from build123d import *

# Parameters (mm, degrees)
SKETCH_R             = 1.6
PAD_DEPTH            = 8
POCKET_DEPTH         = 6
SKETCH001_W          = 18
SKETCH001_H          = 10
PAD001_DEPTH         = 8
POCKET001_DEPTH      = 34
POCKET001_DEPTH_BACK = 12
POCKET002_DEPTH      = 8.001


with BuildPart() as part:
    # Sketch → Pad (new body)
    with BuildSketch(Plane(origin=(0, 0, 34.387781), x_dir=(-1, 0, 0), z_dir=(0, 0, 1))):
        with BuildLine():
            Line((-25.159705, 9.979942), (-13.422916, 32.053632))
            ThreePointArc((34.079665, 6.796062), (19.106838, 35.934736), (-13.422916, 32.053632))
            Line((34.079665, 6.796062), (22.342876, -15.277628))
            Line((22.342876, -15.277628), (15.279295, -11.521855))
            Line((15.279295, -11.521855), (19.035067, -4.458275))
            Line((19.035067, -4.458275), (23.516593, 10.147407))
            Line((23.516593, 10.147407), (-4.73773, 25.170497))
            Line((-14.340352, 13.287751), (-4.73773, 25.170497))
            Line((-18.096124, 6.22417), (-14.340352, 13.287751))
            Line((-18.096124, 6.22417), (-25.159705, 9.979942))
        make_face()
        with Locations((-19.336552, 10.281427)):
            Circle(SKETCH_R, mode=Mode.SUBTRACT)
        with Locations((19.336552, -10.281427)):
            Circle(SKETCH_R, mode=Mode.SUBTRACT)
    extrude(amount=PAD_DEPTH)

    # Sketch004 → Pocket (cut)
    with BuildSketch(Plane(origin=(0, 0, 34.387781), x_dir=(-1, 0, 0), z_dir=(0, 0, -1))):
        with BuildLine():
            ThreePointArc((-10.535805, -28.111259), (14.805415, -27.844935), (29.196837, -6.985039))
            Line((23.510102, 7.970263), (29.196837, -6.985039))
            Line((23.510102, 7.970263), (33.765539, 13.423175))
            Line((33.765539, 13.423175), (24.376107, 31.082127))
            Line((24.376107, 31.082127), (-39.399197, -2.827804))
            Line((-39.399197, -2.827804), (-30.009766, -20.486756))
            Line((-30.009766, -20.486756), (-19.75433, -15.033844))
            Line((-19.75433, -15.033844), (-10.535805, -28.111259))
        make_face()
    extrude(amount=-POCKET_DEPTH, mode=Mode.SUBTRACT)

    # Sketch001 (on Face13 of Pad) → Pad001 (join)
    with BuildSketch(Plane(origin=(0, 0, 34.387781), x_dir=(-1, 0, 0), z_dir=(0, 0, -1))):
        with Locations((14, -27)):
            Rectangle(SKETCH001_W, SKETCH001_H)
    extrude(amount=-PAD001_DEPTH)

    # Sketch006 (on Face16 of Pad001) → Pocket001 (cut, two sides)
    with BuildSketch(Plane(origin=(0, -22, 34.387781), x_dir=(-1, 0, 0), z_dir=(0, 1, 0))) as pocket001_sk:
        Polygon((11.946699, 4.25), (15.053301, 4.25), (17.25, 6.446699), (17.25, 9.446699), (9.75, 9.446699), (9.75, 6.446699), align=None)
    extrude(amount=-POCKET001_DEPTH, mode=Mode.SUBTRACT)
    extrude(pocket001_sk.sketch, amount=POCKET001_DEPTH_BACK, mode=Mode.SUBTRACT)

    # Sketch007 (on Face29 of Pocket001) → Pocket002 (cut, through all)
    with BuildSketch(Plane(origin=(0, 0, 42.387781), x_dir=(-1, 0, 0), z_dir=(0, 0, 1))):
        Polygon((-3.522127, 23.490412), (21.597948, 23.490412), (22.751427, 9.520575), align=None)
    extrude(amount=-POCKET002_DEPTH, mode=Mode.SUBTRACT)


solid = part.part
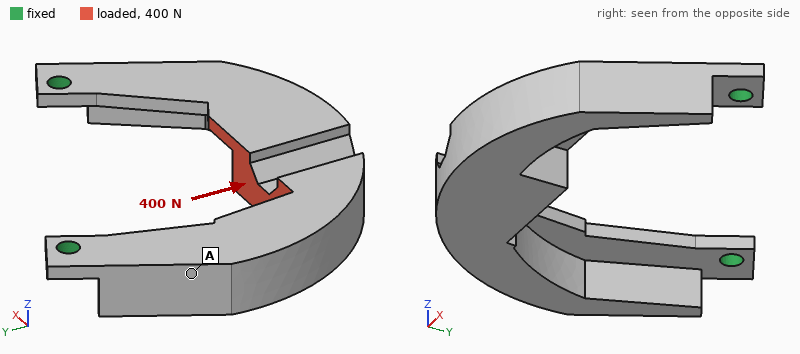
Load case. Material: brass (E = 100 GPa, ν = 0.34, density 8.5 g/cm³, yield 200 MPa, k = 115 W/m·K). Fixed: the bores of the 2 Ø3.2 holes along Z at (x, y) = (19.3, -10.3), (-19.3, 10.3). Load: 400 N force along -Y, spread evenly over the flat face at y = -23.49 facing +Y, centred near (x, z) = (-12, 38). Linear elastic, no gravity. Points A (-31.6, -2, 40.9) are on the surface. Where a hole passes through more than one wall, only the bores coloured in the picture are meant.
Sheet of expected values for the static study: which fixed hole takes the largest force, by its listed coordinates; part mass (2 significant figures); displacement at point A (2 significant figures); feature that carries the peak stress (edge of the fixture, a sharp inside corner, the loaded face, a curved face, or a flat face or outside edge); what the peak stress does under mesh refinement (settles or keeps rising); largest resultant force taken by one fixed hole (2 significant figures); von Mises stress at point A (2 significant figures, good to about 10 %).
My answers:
(-19.3, 10.3)
49 g
0.063 mm
edge of the fixture
keeps rising
280 N
18 MPa
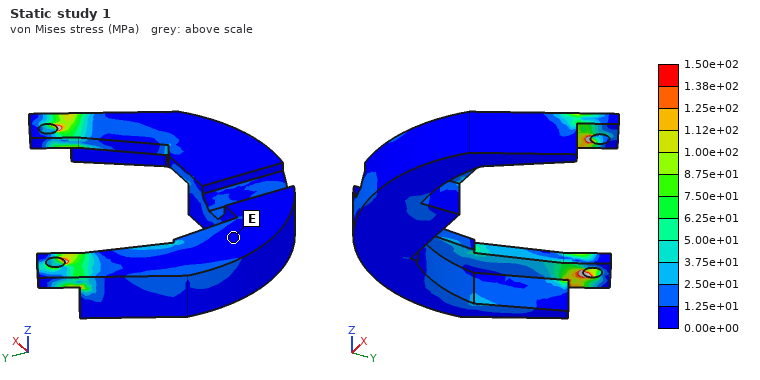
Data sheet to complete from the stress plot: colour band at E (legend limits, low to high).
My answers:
0.00e+00 to 1.25e+01 MPa
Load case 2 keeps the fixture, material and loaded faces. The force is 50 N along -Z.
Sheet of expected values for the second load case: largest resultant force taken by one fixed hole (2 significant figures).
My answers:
26 N
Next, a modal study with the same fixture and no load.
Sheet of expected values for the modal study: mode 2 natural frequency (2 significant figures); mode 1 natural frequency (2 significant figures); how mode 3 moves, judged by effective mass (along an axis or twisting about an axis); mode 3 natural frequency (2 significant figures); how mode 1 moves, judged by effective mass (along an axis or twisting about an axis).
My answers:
2100 Hz
420 Hz
along X
2800 Hz
along Z
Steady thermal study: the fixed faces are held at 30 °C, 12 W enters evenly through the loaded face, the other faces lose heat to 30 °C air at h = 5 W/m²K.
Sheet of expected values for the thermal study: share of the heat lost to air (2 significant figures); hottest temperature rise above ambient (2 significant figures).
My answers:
5.7 %
57 K
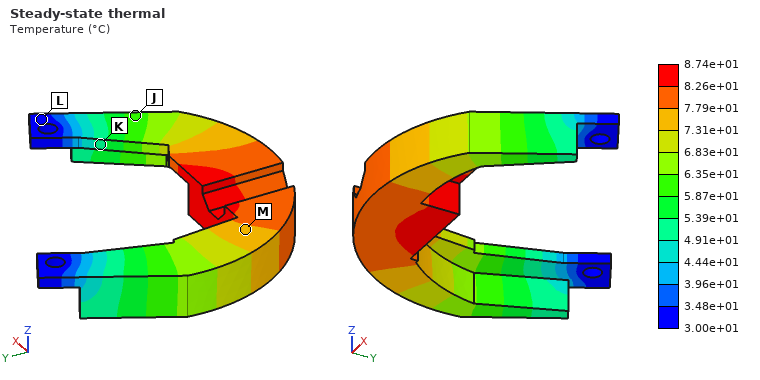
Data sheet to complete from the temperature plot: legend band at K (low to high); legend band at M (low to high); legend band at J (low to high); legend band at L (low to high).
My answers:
4.91e+01 to 5.39e+01 °C
7.31e+01 to 7.79e+01 °C
5.87e+01 to 6.35e+01 °C
3.00e+01 to 3.48e+01 °C
